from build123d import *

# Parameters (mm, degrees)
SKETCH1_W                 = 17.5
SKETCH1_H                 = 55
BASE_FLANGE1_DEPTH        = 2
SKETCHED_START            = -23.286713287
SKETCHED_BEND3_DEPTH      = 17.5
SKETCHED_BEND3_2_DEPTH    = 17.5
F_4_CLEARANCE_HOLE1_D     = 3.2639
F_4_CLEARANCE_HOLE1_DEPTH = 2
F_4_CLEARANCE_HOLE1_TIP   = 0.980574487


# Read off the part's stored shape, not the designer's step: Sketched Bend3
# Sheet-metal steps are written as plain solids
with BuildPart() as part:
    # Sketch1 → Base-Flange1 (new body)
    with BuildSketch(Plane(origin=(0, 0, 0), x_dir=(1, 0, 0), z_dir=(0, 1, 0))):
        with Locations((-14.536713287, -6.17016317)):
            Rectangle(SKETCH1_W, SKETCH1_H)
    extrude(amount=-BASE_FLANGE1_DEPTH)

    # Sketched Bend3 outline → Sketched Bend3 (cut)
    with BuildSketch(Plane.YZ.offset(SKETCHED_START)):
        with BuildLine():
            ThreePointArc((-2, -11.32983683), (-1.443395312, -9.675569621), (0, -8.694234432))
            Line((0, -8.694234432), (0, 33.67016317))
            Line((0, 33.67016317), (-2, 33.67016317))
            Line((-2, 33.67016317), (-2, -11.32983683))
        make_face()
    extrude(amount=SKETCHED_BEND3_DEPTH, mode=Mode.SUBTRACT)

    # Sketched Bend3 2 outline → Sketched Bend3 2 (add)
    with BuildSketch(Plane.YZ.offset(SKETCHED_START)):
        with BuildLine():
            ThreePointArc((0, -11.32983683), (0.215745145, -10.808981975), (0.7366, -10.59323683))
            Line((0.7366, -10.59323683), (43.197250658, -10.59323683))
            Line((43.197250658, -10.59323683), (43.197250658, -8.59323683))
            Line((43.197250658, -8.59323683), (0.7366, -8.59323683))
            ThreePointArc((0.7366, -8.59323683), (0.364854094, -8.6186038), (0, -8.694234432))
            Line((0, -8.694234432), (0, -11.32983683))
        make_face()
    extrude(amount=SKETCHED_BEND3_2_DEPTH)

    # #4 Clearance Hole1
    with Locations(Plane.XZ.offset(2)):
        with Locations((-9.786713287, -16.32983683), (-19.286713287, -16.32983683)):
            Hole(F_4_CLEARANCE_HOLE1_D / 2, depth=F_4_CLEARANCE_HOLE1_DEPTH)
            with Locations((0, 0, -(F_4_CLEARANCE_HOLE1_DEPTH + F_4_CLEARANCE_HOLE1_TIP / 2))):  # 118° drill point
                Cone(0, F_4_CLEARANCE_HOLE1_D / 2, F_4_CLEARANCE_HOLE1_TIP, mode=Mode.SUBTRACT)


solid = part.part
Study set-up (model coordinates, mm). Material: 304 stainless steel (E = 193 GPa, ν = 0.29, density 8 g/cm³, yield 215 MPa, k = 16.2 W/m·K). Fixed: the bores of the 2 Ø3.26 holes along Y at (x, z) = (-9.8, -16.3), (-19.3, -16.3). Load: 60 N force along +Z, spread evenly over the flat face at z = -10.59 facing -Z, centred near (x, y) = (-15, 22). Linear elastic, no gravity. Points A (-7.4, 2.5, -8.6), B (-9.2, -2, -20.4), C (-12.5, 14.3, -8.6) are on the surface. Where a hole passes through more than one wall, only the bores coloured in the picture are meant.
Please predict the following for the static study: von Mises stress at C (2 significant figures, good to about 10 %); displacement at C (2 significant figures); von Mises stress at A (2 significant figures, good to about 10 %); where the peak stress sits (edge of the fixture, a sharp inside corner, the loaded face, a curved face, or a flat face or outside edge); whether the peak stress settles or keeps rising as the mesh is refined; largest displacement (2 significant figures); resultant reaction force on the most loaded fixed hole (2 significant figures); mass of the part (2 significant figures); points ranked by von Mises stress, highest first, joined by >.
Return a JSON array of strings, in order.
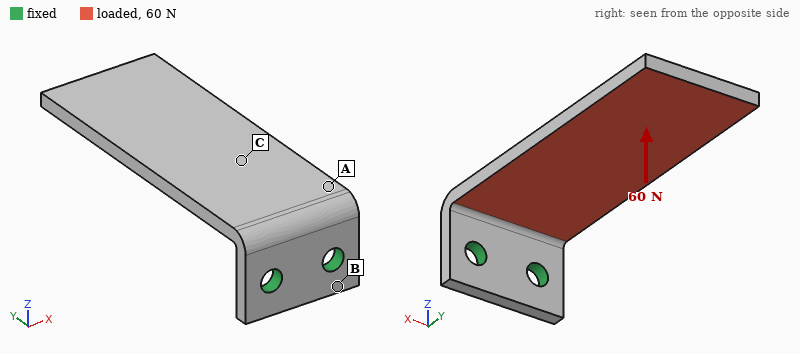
["49 MPa", "0.10 mm", "99 MPa", "edge of the fixture", "keeps rising", "0.42 mm", "37 N", "15 g", "A > C > B"]
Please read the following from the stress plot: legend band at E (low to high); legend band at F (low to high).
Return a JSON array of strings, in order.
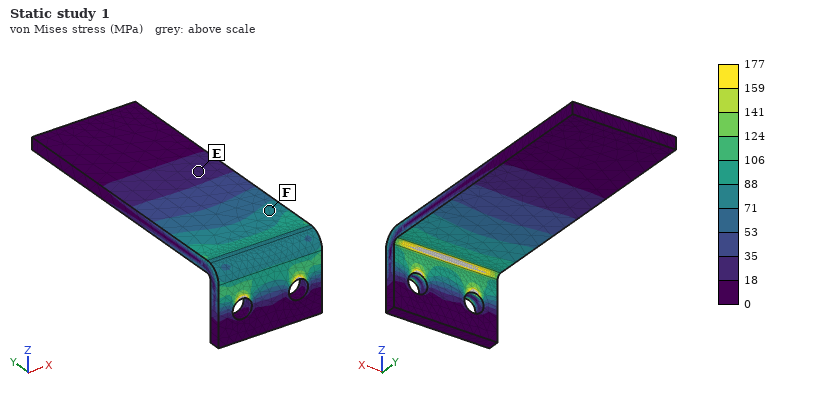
["18 to 35 MPa", "71 to 88 MPa"]
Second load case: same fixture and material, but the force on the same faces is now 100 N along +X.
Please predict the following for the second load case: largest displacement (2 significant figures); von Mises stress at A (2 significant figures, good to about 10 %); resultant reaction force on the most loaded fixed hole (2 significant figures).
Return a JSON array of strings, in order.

["65 µm", "31 MPa", "210 N"]
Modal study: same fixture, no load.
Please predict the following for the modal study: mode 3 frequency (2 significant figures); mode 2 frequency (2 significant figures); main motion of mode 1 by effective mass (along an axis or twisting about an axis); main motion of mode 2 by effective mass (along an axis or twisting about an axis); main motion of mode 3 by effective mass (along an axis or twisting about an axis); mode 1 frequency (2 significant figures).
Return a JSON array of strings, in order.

["4200 Hz", "2300 Hz", "along Z", "along X", "twisting about Y", "680 Hz"]
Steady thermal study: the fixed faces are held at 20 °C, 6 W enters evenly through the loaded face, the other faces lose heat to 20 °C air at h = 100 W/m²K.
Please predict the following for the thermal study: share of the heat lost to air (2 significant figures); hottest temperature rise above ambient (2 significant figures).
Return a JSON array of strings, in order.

["77 %", "56 K"]
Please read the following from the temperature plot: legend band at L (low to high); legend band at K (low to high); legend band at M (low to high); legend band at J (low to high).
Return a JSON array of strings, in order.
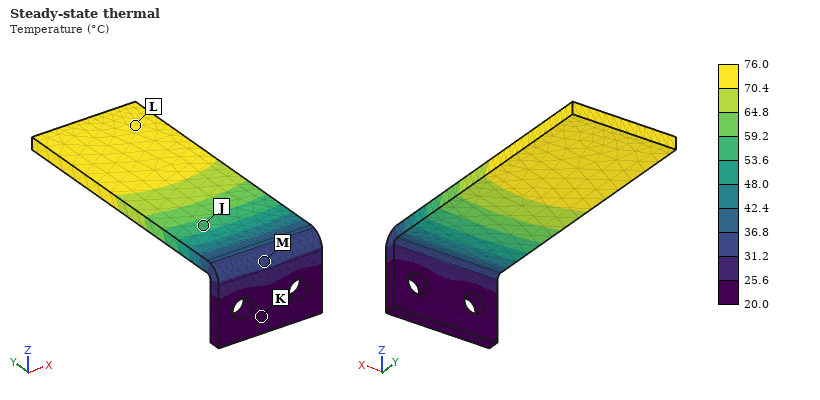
["70.4 to 76.0 °C", "20.0 to 25.6 °C", "31.2 to 36.8 °C", "53.6 to 59.2 °C"]
